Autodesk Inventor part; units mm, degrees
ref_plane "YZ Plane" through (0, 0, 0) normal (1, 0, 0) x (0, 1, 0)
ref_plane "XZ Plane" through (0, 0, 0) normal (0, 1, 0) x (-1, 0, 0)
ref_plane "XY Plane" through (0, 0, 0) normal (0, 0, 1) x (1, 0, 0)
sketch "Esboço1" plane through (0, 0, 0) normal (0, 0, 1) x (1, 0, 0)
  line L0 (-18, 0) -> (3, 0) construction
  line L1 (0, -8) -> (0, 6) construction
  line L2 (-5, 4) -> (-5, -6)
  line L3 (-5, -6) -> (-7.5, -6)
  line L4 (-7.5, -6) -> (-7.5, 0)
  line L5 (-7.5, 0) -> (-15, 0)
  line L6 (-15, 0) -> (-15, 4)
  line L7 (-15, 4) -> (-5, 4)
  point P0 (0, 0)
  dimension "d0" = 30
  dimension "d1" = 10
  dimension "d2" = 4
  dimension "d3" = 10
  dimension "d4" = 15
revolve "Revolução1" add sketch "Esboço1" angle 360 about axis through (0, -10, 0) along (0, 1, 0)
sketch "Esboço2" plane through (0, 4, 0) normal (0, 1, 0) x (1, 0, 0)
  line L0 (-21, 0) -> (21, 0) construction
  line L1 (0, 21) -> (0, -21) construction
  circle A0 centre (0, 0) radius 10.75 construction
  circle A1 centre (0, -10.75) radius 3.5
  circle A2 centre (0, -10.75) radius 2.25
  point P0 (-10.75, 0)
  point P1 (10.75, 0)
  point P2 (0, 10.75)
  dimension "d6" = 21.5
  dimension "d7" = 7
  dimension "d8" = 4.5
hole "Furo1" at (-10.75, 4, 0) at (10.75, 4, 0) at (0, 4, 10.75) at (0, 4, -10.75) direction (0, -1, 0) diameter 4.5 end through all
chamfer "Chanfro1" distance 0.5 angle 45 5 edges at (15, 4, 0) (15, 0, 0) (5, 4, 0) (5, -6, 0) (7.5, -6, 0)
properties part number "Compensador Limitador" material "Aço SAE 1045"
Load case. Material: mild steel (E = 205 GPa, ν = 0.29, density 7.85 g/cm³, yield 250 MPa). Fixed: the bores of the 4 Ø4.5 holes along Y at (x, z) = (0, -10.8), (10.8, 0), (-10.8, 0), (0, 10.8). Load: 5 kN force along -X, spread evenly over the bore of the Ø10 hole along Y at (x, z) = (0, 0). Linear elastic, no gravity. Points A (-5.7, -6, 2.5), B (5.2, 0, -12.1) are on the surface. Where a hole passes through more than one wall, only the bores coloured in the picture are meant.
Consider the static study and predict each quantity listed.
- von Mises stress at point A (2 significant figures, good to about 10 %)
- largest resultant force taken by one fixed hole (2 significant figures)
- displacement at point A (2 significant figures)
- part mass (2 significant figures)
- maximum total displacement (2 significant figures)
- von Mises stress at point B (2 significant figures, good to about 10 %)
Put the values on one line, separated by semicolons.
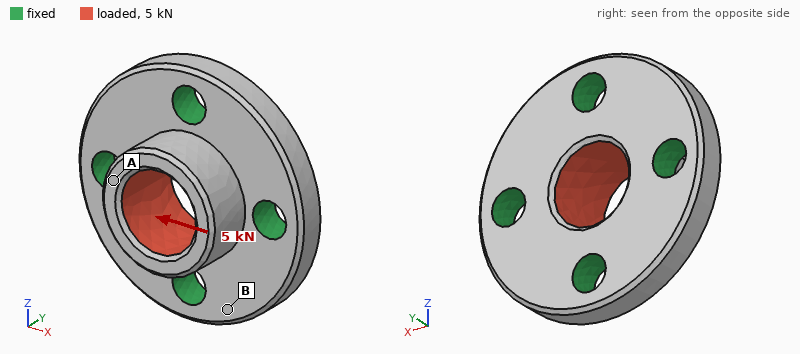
44 MPa; 1.6 kN; 4.7 µm; 22 g; 4.8 µm; 9.9 MPa
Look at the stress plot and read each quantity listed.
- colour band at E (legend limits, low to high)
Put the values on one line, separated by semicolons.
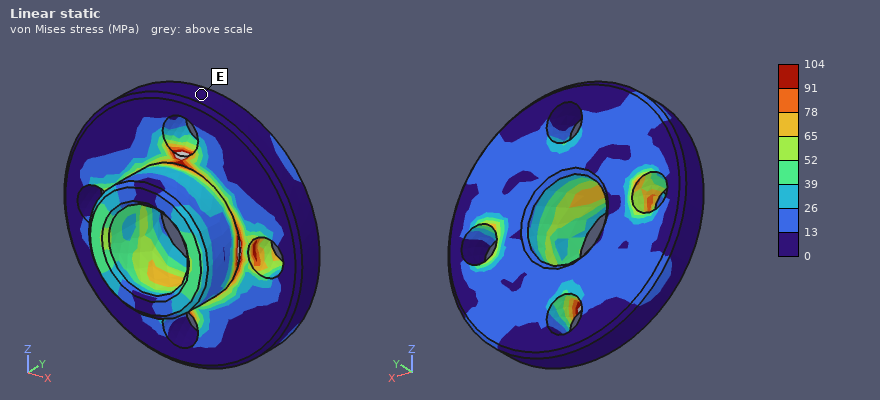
0 to 13 MPa
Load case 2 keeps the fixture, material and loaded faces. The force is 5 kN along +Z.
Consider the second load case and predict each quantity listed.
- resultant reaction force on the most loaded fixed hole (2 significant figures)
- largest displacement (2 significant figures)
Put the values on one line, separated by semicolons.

1.6 kN; 4.8 µm
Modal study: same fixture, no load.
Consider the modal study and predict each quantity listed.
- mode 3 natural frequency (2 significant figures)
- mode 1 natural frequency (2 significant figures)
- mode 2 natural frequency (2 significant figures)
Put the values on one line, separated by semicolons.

61 kHz; 59 kHz; 61 kHz
